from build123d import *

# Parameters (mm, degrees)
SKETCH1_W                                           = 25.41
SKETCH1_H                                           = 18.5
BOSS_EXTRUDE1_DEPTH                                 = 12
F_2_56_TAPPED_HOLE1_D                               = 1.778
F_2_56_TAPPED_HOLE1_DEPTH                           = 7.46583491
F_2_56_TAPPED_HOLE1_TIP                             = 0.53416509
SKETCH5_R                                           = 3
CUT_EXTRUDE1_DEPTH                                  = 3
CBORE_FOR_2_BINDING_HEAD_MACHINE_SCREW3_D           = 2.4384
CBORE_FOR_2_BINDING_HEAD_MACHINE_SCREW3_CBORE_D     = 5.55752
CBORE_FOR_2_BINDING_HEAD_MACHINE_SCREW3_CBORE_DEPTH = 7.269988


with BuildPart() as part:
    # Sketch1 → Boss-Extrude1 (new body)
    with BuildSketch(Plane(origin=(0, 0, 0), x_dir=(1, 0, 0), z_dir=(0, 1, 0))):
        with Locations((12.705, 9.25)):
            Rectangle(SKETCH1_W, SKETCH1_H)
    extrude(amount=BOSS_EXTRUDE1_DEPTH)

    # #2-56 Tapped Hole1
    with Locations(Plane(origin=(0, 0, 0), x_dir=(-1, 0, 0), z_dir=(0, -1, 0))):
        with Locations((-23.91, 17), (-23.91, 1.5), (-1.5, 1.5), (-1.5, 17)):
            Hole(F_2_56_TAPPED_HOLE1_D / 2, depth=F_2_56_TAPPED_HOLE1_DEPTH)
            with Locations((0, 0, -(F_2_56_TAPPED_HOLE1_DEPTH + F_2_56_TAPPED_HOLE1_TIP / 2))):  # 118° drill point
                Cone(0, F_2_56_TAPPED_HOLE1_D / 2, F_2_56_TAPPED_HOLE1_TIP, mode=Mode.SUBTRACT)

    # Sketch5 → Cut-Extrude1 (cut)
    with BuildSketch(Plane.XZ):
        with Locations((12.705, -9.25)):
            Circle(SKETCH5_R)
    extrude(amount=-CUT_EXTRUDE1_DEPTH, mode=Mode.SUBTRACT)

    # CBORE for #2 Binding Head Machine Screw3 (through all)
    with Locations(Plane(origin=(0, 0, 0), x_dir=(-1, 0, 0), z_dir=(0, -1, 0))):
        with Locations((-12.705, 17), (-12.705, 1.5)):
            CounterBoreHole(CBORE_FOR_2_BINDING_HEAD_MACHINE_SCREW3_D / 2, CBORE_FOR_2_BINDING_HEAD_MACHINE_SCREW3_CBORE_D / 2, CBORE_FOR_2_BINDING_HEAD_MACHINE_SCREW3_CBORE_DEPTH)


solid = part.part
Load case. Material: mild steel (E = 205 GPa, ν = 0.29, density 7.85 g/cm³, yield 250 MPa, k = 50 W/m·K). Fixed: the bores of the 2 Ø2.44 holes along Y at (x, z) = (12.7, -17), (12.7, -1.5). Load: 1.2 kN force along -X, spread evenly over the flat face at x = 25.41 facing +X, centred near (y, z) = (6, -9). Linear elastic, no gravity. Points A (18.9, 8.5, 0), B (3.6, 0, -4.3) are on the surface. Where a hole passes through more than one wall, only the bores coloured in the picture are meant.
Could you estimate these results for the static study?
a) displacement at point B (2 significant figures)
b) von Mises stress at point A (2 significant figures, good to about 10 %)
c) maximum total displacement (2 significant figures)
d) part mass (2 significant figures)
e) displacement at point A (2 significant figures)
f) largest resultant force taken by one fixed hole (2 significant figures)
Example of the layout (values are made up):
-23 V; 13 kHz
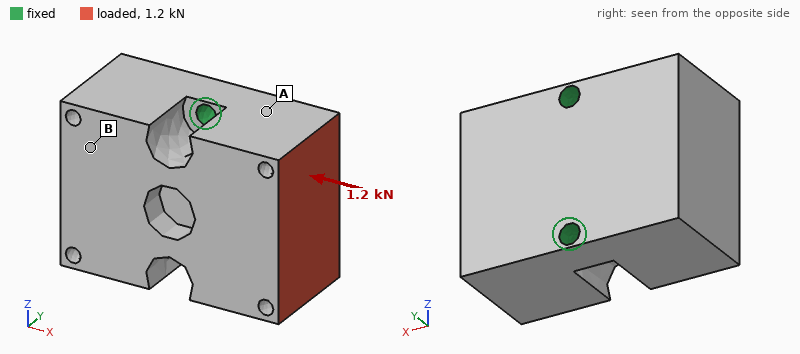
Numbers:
4.1 µm; 16 MPa; 5.7 µm; 40 g; 1.8 µm; 600 N
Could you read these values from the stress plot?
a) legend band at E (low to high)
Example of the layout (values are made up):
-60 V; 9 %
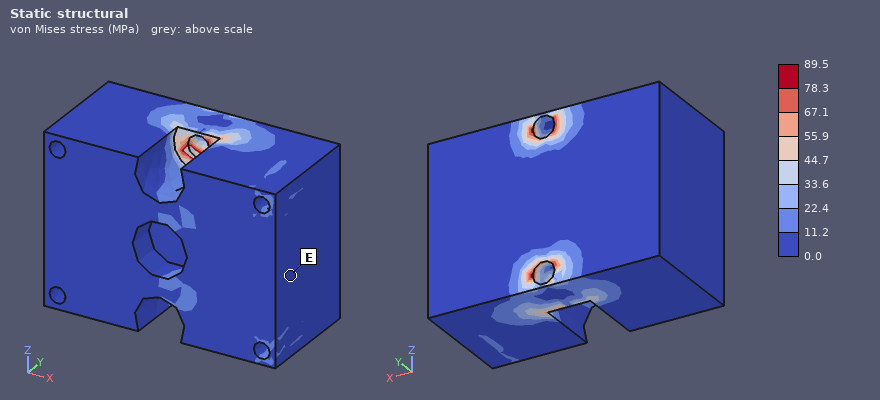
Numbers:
0.0 to 11.2 MPa
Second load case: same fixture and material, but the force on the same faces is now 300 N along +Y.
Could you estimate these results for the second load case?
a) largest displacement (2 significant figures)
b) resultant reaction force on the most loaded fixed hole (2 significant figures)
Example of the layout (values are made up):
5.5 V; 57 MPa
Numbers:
4.8 µm; 160 N
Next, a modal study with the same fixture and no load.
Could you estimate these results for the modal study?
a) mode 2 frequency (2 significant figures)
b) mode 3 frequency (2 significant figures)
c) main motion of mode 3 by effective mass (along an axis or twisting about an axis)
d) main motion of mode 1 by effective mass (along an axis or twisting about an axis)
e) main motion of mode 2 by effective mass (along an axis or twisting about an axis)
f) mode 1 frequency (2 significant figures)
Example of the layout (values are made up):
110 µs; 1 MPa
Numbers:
28 kHz; 29 kHz; along Z; along X; along Y; 11 kHz
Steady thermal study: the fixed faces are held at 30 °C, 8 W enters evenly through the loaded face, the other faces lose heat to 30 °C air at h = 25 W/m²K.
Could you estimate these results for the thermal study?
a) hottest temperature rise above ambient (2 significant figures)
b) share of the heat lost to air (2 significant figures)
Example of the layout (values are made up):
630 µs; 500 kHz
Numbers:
15 K; 4.1 %
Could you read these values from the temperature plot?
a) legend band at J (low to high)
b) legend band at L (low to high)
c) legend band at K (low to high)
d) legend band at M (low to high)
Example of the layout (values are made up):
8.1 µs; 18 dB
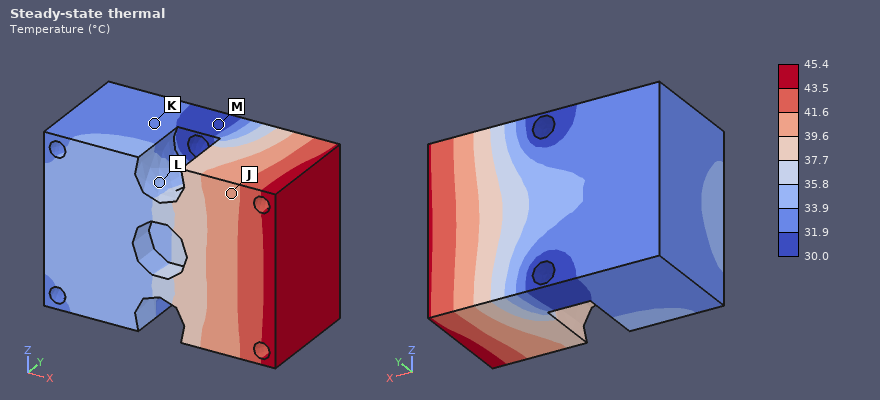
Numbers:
39.6 to 41.6 °C; 33.9 to 35.8 °C; 31.9 to 33.9 °C; 30.0 to 31.9 °C
